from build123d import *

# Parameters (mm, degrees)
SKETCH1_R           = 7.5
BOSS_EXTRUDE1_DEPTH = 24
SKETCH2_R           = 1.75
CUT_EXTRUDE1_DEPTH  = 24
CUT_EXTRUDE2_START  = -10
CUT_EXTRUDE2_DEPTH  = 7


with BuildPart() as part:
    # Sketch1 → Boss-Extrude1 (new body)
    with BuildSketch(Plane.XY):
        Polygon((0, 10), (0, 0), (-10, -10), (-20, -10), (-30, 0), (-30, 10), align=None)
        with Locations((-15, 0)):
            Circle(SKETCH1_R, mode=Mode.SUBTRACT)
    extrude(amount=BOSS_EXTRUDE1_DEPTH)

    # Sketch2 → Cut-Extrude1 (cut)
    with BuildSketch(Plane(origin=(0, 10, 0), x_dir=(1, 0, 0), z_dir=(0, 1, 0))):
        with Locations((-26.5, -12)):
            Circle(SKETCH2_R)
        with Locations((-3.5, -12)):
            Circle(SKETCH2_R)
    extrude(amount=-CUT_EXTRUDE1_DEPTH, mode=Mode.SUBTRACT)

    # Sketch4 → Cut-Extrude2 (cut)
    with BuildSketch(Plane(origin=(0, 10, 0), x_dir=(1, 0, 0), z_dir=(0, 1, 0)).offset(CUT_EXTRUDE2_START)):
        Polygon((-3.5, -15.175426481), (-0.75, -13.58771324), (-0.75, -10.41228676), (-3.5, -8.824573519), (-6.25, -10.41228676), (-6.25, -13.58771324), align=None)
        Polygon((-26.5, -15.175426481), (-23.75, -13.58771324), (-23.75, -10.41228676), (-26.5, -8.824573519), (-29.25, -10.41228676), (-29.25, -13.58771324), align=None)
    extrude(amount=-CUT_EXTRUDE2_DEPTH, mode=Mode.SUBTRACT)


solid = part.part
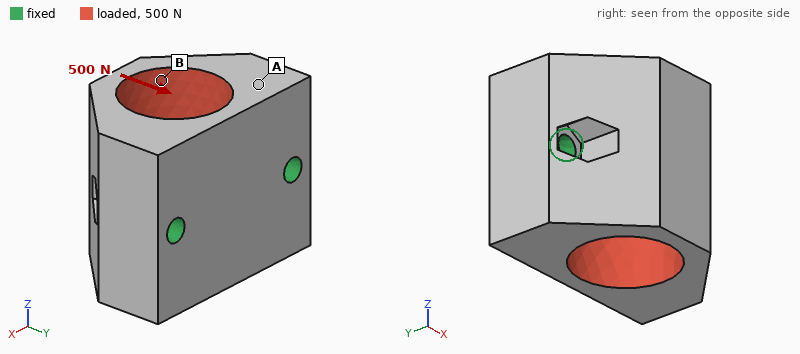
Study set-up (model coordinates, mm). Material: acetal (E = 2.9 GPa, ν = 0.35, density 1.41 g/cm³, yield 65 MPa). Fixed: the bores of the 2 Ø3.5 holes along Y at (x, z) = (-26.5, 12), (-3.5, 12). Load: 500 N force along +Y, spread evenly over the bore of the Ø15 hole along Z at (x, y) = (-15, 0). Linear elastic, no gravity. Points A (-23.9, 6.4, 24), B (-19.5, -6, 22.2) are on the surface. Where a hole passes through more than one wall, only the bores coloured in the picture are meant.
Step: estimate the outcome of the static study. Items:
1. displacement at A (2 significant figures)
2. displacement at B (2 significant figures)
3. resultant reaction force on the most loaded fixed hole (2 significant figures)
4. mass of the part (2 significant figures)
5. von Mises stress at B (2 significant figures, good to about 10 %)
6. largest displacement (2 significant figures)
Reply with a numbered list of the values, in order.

1. 13 µm
2. 16 µm
3. 250 N
4. 10 g
5. 2.0 MPa
6. 23 µm
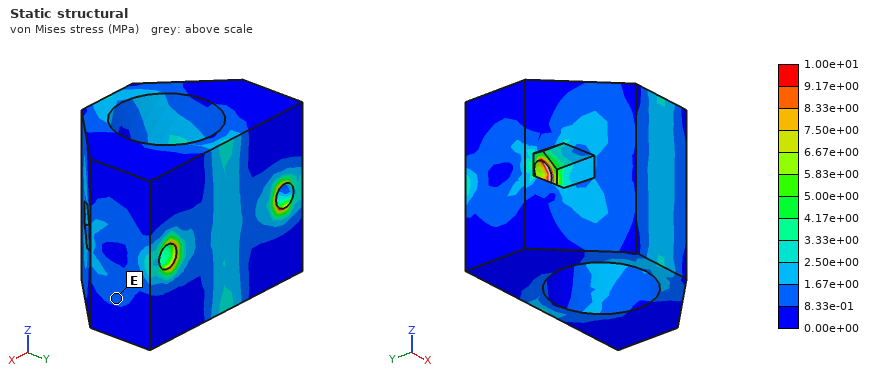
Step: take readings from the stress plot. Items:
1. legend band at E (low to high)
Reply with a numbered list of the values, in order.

1. 8.33e-01 to 1.67e+00 MPa
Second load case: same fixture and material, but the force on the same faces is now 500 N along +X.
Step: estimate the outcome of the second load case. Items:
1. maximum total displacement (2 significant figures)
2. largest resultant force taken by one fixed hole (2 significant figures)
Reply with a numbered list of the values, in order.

1. 38 µm
2. 260 N
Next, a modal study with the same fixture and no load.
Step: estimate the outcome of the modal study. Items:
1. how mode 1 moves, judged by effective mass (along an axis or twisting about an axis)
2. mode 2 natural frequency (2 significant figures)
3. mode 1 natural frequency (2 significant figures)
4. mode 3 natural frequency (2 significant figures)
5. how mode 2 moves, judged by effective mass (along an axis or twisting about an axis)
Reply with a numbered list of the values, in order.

1. along Z
2. 7800 Hz
3. 6100 Hz
4. 9400 Hz
5. along X
